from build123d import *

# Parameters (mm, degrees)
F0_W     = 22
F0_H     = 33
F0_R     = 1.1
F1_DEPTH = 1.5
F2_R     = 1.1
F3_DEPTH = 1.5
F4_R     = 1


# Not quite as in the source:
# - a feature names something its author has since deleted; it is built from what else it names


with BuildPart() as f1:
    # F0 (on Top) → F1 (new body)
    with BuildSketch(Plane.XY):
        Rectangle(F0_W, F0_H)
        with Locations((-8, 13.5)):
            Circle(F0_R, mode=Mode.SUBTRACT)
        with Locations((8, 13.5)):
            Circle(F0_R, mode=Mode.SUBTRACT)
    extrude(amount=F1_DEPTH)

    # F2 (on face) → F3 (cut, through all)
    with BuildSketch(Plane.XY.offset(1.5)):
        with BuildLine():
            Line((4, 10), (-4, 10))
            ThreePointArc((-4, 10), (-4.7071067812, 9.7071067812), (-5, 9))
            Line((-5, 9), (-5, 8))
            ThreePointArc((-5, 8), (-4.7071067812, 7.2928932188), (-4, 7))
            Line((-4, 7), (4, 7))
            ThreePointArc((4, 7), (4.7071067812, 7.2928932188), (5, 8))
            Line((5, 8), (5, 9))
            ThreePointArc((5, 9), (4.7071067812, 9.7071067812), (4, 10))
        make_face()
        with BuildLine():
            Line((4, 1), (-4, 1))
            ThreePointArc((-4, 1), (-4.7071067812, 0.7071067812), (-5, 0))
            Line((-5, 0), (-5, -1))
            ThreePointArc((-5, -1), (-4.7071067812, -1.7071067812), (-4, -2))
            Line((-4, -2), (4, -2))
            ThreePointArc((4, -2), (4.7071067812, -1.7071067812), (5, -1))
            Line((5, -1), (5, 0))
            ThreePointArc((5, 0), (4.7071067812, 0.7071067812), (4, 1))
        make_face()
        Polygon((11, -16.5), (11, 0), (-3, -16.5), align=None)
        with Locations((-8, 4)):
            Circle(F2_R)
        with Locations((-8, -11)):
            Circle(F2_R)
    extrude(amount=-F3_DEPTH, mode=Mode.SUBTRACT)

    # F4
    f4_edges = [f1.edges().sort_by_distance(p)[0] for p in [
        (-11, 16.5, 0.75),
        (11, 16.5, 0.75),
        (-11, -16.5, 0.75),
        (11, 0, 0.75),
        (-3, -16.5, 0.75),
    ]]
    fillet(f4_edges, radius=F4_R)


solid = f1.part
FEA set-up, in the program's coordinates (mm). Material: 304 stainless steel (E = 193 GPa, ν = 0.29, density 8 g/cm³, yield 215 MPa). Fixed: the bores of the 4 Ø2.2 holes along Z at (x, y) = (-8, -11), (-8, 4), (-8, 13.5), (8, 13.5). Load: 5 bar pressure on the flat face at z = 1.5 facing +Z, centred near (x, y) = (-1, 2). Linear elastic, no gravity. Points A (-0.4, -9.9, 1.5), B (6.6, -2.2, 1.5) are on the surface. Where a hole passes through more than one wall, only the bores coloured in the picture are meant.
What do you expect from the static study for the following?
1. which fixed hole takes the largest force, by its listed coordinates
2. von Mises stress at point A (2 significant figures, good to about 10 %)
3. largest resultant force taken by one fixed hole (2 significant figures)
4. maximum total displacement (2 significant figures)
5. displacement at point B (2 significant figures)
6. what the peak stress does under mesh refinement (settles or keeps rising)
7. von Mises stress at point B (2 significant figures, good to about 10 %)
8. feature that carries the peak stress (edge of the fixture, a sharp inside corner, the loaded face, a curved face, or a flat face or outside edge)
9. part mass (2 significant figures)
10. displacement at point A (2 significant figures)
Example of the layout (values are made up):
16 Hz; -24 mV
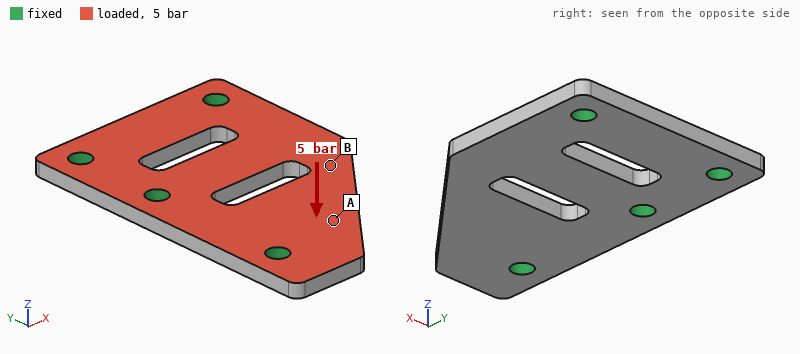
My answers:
(-8, -11); 15 MPa; 88 N; 30 µm; 25 µm; keeps rising; 45 MPa; edge of the fixture; 6.4 g; 11 µm
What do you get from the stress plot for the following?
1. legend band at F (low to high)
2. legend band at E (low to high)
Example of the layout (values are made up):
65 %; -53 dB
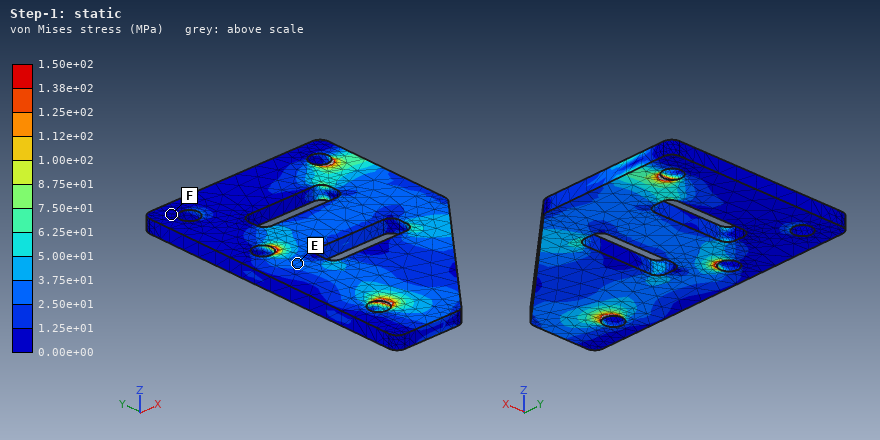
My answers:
0.00e+00 to 1.25e+01 MPa; 2.50e+01 to 3.75e+01 MPa
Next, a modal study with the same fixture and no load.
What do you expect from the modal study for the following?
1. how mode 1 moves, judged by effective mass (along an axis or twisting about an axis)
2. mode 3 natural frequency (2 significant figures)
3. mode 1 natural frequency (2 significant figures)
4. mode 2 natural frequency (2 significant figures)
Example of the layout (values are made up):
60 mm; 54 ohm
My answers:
along Z; 25 kHz; 7900 Hz; 18 kHz
